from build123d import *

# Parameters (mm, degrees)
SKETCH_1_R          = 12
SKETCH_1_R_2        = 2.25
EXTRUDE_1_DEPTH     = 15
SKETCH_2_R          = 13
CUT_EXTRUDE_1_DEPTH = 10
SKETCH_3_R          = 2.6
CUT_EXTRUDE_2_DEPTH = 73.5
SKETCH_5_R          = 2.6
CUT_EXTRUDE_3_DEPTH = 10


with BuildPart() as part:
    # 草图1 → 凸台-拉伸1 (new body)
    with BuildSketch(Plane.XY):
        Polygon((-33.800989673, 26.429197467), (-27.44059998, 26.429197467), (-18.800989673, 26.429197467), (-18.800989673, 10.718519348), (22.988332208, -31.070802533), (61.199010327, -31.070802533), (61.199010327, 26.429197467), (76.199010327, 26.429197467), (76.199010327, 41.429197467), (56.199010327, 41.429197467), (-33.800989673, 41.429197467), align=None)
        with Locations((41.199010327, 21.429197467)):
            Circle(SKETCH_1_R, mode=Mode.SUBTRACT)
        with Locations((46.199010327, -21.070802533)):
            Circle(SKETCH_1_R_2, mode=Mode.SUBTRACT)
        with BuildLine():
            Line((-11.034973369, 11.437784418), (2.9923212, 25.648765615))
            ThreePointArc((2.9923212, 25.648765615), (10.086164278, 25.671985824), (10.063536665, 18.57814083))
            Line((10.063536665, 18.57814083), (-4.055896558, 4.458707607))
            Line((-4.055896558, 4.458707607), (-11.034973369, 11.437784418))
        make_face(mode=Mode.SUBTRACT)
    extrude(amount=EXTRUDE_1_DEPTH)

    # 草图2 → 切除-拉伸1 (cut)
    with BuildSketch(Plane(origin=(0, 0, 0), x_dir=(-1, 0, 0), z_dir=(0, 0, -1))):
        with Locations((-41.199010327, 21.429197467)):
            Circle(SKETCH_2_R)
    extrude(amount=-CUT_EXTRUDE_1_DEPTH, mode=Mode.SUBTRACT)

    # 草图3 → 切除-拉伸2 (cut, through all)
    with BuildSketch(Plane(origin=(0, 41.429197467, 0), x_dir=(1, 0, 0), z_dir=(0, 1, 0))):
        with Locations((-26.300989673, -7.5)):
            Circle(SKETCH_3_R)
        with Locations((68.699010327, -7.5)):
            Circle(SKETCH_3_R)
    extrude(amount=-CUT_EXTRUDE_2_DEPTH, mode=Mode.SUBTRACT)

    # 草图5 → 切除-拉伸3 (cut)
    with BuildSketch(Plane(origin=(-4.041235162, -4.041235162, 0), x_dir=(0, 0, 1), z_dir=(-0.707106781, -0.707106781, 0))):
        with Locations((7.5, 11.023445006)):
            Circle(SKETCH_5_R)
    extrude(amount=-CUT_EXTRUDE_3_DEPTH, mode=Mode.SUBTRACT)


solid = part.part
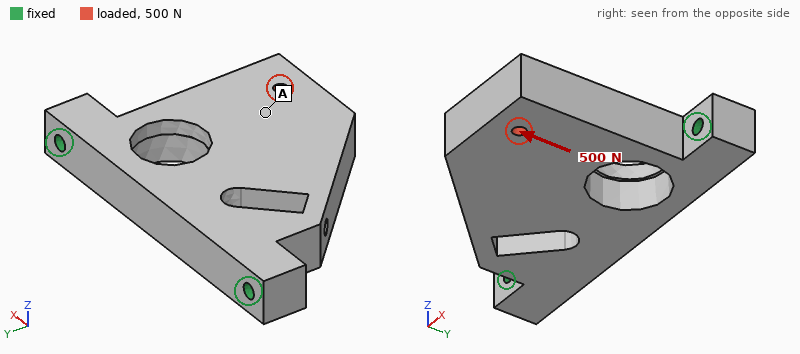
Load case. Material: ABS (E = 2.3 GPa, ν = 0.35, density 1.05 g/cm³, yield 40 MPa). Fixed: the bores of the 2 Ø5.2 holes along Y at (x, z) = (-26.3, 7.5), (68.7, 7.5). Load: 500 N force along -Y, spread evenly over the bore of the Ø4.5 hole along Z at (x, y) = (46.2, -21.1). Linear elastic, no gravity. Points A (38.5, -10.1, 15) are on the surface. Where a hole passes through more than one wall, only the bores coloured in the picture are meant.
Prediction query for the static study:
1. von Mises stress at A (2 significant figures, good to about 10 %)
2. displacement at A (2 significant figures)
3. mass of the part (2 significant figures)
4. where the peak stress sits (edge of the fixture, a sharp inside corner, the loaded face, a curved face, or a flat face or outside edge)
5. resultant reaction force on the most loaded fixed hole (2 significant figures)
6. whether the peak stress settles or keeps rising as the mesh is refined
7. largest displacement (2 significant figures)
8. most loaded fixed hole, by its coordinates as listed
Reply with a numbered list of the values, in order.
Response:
1. 0.75 MPa
2. 64 µm
3. 72 g
4. edge of the fixture
5. 400 N
6. keeps rising
7. 85 µm
8. (68.7, 7.5)
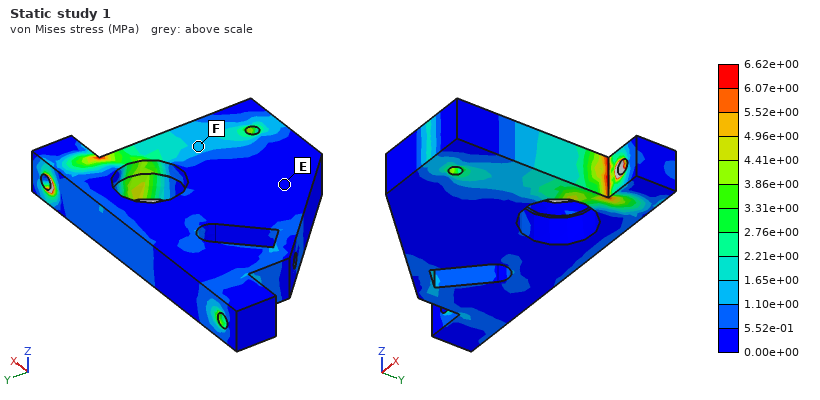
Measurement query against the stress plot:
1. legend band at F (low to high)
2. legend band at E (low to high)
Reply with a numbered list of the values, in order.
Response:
1. 1.10e+00 to 1.65e+00 MPa
2. 0.00e+00 to 5.52e-01 MPa
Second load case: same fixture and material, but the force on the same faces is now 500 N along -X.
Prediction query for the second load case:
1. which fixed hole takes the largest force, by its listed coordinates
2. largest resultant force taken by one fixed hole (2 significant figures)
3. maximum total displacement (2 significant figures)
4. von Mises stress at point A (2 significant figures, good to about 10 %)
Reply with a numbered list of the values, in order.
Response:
1. (-26.3, 7.5)
2. 460 N
3. 0.17 mm
4. 1.5 MPa
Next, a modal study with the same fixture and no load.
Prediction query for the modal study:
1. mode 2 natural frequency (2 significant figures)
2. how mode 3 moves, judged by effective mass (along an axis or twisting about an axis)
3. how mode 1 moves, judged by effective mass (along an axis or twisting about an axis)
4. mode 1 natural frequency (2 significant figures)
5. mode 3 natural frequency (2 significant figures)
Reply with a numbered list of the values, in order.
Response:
1. 1500 Hz
2. along X
3. along Z
4. 430 Hz
5. 1800 Hz
